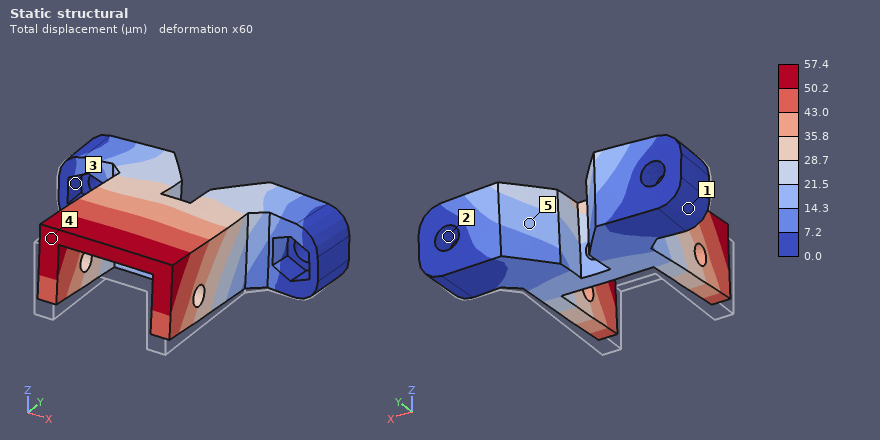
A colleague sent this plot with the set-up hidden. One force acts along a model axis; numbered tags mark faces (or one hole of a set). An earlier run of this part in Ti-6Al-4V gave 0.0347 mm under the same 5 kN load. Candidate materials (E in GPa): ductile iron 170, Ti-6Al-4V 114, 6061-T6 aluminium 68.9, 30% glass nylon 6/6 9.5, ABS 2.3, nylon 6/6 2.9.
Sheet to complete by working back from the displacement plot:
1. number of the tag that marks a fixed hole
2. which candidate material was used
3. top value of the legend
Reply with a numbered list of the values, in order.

1. 2
2. 6061-T6 aluminium
3. 57.4 µm
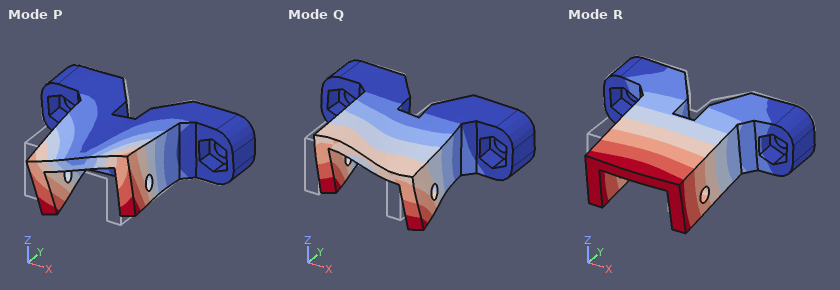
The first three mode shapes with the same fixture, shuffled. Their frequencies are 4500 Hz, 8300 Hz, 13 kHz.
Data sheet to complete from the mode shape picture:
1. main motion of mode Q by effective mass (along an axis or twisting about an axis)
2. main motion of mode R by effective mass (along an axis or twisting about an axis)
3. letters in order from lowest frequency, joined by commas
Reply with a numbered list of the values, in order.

1. along X
2. along Z
3. R, P, Q
